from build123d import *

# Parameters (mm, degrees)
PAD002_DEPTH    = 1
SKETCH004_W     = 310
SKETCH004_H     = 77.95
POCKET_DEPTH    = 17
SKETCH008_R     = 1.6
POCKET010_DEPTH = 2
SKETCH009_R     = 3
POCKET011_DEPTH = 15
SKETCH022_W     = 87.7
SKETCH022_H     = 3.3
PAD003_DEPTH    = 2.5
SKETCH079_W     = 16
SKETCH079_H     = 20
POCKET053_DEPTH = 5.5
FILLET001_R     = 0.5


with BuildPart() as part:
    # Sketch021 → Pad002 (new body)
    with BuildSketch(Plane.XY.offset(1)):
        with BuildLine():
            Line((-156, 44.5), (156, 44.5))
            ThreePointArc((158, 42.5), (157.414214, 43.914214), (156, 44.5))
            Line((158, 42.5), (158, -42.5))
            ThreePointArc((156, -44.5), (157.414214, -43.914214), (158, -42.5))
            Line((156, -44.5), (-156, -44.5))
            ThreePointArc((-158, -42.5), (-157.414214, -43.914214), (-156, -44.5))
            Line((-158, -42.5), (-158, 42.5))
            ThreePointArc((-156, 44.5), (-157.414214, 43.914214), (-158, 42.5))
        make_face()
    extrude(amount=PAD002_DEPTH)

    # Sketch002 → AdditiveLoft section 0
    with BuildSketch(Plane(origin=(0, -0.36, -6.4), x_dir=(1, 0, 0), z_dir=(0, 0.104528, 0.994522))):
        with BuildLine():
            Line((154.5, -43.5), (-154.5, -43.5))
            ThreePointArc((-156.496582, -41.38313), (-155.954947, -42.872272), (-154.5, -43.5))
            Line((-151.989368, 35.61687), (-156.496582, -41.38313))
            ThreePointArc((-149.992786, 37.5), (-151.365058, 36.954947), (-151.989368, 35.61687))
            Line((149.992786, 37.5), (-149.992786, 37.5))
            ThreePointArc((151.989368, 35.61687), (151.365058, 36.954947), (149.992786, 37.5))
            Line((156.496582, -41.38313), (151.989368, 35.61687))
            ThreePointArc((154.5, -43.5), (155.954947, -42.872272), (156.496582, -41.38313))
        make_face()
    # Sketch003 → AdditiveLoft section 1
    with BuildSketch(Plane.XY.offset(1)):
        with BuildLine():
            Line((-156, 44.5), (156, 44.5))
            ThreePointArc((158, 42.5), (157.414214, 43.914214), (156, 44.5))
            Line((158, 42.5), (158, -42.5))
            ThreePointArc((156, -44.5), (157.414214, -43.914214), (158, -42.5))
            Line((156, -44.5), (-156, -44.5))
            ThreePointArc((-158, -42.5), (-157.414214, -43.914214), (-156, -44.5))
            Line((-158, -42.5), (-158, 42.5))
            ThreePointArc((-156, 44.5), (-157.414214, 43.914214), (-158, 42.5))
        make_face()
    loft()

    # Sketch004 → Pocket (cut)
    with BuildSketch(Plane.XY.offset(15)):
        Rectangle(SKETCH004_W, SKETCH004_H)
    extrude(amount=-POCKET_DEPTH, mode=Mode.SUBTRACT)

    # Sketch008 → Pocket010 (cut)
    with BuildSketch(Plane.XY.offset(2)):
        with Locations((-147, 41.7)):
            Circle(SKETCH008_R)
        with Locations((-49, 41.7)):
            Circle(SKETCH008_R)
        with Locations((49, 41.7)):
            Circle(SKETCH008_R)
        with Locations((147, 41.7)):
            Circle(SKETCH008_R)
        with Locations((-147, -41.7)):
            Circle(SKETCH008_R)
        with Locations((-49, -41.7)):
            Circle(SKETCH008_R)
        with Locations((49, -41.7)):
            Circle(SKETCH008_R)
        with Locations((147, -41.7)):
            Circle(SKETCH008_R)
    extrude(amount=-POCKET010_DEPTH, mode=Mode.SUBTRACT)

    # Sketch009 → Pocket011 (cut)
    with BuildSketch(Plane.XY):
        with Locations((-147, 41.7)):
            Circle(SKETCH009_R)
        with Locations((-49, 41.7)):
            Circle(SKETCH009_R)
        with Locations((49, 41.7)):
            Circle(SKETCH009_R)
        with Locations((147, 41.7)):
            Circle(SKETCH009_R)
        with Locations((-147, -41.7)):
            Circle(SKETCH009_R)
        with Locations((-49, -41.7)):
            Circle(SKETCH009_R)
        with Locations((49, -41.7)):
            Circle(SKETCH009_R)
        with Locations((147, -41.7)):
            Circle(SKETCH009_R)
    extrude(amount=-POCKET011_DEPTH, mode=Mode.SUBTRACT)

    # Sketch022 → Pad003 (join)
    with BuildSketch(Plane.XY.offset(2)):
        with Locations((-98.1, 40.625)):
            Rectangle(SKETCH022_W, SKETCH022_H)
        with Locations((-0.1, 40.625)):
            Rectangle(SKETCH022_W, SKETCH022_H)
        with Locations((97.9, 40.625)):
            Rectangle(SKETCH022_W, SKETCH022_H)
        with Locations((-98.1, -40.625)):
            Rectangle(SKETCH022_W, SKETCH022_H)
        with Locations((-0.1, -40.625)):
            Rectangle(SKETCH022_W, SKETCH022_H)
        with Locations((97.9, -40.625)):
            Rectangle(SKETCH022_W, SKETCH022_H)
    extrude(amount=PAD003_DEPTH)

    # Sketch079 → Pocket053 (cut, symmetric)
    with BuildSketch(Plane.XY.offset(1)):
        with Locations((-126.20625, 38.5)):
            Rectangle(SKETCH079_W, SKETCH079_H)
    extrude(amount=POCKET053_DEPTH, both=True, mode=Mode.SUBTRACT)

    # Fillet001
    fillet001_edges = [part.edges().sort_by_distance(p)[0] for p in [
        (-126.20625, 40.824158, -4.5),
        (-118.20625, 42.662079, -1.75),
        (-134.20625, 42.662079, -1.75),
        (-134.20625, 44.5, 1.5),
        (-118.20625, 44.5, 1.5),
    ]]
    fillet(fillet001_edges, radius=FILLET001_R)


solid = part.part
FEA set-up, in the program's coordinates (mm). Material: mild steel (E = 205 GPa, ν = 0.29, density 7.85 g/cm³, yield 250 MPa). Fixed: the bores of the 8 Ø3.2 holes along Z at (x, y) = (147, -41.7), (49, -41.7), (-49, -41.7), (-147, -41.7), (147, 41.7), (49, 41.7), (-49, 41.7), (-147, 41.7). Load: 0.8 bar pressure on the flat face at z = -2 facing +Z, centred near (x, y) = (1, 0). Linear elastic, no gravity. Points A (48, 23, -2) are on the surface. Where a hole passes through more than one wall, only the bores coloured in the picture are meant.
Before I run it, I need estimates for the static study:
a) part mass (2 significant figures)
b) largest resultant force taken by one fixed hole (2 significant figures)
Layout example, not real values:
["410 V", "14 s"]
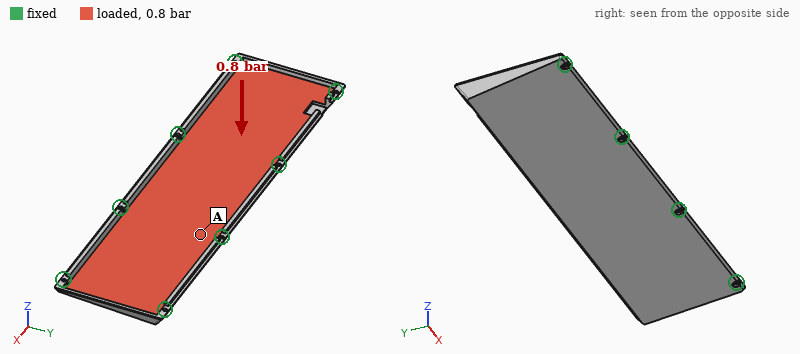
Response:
["990 g", "680 N"]
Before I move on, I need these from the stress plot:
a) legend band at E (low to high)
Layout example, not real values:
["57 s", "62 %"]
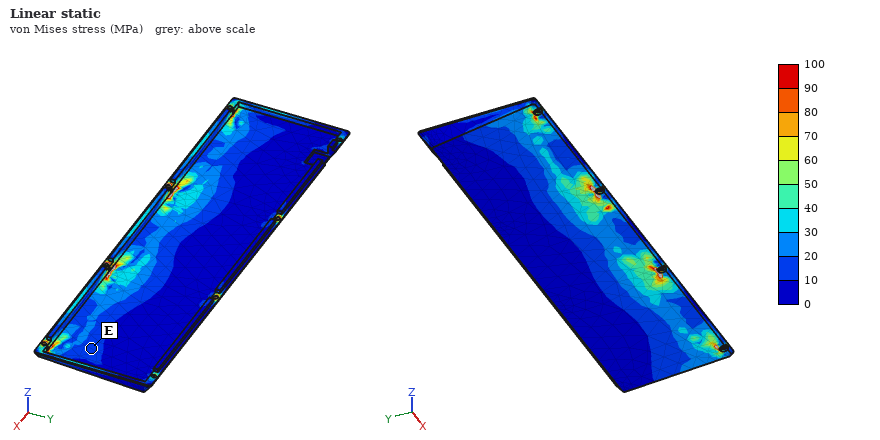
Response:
["10 to 20 MPa"]
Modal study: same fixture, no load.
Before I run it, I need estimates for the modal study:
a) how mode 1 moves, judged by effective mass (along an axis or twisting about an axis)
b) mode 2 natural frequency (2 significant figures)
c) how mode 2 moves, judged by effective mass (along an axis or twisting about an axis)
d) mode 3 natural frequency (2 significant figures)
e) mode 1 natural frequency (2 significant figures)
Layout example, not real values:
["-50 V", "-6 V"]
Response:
["along Z", "1600 Hz", "twisting about Y", "1800 Hz", "1400 Hz"]
